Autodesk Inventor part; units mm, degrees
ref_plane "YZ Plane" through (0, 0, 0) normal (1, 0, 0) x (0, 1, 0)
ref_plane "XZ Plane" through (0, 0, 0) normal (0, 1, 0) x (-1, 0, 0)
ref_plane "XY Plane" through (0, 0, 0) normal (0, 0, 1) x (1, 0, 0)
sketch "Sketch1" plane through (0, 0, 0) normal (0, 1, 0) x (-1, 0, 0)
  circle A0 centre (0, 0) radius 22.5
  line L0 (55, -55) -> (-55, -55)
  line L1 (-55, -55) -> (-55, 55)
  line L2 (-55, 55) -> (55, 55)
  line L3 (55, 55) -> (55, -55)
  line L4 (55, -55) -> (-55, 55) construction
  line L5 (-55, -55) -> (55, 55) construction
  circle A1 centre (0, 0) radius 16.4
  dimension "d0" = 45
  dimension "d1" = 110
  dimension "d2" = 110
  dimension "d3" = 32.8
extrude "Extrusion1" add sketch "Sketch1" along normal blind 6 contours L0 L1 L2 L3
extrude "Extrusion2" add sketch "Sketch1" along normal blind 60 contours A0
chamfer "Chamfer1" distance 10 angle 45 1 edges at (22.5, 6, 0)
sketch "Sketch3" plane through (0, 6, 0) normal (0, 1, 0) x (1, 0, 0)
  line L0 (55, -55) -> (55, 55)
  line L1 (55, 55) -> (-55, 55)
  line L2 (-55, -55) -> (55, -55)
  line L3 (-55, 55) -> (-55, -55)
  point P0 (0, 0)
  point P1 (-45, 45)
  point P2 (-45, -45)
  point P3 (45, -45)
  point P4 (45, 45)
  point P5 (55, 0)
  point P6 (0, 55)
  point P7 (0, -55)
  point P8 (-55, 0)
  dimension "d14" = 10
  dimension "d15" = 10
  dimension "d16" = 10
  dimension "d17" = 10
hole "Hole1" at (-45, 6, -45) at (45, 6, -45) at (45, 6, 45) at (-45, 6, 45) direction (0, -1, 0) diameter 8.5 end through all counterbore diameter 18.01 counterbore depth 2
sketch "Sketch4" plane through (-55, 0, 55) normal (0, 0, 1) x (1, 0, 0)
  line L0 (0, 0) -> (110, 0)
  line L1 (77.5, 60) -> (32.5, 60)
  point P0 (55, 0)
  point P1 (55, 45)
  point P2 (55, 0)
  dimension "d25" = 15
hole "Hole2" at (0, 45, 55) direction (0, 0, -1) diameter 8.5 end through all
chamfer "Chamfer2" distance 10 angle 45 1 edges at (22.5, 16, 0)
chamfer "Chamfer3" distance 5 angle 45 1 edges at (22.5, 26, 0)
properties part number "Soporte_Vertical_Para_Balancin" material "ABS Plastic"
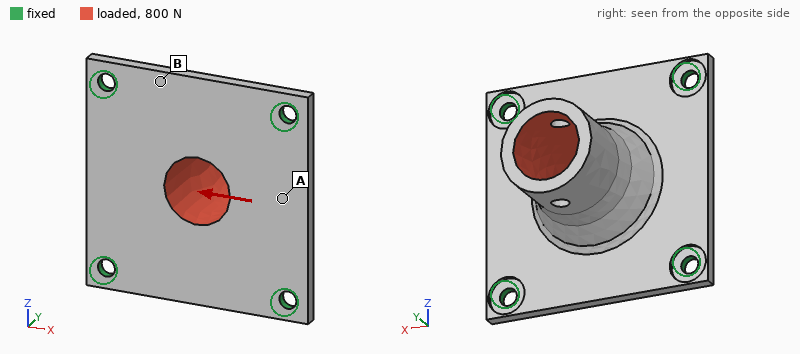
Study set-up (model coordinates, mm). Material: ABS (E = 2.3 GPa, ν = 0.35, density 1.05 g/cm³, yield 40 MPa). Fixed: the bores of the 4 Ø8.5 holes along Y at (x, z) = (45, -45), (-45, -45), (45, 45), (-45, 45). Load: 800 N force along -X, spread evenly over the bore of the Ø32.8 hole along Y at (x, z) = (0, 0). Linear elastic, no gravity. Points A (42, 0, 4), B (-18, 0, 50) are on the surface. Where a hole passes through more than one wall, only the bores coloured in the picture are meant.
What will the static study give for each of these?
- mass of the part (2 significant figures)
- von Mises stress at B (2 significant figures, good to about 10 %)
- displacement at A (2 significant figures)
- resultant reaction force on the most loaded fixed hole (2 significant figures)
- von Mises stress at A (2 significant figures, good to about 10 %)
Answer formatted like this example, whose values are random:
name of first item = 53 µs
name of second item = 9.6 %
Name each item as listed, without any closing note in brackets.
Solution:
mass of the part = 120 g
von Mises stress at B = 2.0 MPa
displacement at A = 0.37 mm
resultant reaction force on the most loaded fixed hole = 300 N
von Mises stress at A = 4.0 MPa
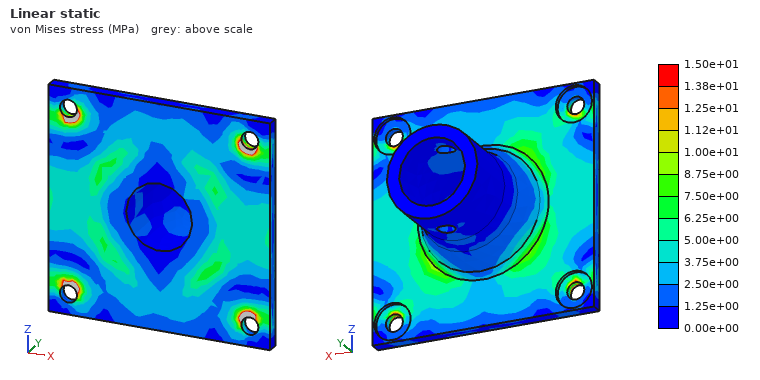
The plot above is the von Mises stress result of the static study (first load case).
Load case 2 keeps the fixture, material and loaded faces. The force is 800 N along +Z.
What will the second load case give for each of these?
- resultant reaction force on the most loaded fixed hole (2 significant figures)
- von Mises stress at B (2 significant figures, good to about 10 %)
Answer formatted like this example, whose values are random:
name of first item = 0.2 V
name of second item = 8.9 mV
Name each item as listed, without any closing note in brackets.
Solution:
resultant reaction force on the most loaded fixed hole = 300 N
von Mises stress at B = 3.1 MPa
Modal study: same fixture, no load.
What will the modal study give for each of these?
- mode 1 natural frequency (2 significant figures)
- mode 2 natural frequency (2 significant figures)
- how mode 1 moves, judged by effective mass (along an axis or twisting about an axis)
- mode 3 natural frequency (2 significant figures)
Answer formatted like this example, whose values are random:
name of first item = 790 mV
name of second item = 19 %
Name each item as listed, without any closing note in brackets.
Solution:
mode 1 natural frequency = 620 Hz
mode 2 natural frequency = 750 Hz
how mode 1 moves, judged by effective mass = along Y
mode 3 natural frequency = 750 Hz
